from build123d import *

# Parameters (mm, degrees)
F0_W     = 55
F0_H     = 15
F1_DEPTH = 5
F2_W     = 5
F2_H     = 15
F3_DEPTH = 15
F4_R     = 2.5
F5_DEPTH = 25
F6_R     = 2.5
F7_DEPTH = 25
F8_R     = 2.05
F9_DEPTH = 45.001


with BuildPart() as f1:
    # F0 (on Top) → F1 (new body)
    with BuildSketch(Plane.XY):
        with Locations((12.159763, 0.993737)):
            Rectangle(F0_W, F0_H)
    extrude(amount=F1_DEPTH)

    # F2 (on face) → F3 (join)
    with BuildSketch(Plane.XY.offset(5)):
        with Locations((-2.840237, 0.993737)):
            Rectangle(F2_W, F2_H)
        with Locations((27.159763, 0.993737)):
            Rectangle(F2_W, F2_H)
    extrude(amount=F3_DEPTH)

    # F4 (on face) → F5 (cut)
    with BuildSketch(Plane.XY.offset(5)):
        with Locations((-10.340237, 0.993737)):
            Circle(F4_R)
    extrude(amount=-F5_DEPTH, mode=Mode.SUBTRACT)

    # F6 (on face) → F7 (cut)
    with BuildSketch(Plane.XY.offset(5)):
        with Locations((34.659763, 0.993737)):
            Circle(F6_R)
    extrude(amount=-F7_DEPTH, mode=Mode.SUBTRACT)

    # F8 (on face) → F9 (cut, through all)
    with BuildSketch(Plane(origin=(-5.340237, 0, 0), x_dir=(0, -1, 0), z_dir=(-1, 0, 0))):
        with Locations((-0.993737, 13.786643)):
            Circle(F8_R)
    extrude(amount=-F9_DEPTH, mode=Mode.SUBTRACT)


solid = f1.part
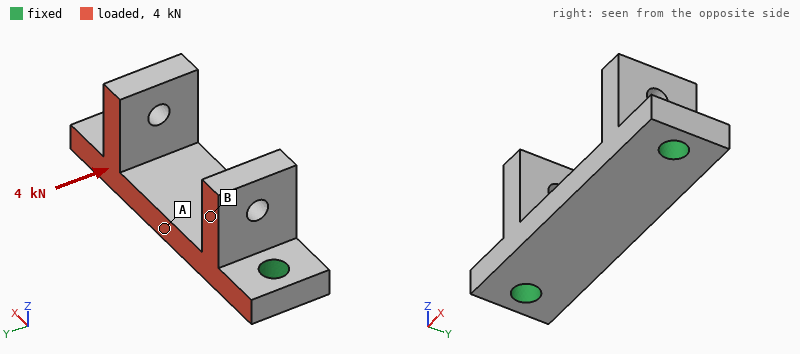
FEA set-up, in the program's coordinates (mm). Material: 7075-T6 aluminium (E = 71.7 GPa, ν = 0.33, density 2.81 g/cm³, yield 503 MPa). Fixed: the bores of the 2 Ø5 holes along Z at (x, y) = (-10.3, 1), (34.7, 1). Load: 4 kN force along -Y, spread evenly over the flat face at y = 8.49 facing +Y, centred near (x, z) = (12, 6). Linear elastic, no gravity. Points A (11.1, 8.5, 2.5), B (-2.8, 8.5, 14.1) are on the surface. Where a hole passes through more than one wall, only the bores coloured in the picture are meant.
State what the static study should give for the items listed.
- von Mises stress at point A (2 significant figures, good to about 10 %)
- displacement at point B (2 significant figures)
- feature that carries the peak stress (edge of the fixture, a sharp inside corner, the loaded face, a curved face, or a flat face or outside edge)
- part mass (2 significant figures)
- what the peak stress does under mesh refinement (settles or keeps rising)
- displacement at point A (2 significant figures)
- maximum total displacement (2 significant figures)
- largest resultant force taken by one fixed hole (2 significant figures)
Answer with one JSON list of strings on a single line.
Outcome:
["39 MPa", "44 µm", "edge of the fixture", "17 g", "keeps rising", "26 µm", "59 µm", "2.0 kN"]
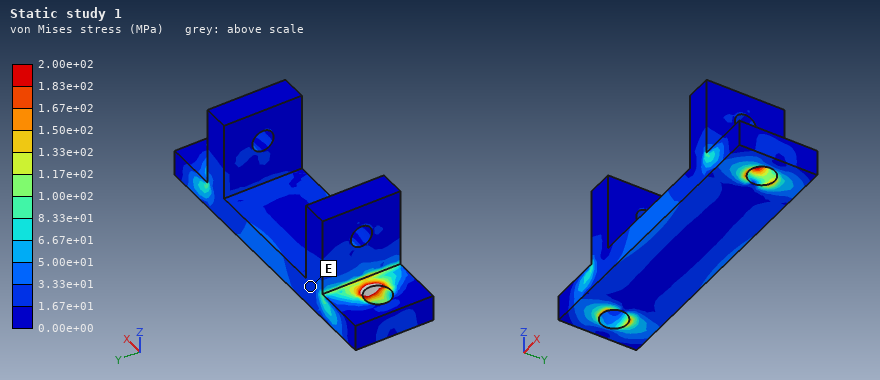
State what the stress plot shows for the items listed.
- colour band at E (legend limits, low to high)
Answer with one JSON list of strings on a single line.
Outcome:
["1.67e+01 to 3.33e+01 MPa"]
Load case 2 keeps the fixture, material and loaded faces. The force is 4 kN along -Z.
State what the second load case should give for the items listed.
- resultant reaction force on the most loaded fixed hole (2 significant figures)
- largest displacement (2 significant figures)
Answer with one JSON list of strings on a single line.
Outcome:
["2.0 kN", "0.12 mm"]
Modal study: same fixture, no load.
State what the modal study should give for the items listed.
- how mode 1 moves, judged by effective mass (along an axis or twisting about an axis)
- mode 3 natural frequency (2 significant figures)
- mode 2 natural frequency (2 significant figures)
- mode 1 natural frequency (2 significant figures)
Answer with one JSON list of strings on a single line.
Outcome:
["along Z", "12 kHz", "12 kHz", "8700 Hz"]
